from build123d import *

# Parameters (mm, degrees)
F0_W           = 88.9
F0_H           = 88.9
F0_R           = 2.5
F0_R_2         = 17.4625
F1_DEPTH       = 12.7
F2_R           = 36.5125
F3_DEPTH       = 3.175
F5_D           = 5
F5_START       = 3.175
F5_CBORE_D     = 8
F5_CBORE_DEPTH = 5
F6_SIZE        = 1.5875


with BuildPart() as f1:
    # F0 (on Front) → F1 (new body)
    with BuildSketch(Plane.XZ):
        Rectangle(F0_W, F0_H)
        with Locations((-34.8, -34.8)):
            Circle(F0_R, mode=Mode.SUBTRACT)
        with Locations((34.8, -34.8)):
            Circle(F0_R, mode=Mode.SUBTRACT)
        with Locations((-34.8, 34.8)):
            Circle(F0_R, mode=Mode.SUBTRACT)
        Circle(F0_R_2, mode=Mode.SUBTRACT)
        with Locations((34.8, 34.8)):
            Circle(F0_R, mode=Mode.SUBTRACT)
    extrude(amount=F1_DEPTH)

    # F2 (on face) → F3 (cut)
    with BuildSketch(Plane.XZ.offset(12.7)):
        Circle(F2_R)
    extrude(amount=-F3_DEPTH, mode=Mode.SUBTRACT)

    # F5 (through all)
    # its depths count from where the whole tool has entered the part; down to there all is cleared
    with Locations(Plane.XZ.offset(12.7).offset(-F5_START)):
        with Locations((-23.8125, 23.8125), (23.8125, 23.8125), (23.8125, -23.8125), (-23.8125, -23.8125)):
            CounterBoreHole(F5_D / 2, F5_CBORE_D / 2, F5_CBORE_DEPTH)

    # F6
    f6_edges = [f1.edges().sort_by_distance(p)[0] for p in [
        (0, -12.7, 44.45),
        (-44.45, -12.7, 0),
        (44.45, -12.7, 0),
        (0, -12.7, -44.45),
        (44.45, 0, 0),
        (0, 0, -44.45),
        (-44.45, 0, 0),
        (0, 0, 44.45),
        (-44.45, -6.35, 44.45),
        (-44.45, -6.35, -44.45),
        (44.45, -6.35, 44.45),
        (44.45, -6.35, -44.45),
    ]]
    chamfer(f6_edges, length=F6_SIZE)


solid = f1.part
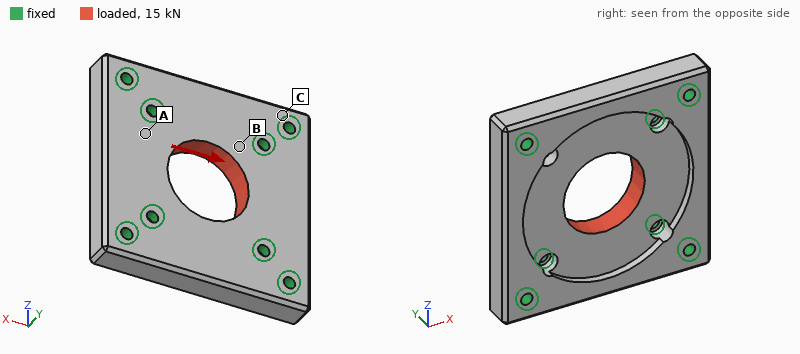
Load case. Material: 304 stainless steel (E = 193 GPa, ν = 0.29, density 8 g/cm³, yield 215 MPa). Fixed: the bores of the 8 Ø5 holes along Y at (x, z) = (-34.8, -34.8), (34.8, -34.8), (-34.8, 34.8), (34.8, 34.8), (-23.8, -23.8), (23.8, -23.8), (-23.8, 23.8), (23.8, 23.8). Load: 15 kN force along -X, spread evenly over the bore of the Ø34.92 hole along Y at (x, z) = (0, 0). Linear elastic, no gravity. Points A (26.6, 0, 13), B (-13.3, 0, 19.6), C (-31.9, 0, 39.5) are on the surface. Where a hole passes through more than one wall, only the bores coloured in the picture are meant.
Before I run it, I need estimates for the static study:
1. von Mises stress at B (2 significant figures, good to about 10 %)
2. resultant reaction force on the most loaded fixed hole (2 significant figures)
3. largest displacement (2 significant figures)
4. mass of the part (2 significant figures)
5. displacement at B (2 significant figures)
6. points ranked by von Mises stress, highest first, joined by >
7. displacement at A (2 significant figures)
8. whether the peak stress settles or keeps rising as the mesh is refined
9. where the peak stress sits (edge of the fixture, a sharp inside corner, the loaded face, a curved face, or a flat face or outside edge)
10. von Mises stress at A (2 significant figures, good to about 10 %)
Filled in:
22 MPa
2.5 kN
3.7 µm
600 g
1.5 µm
B > A > C
1.9 µm
keeps rising
edge of the fixture
13 MPa
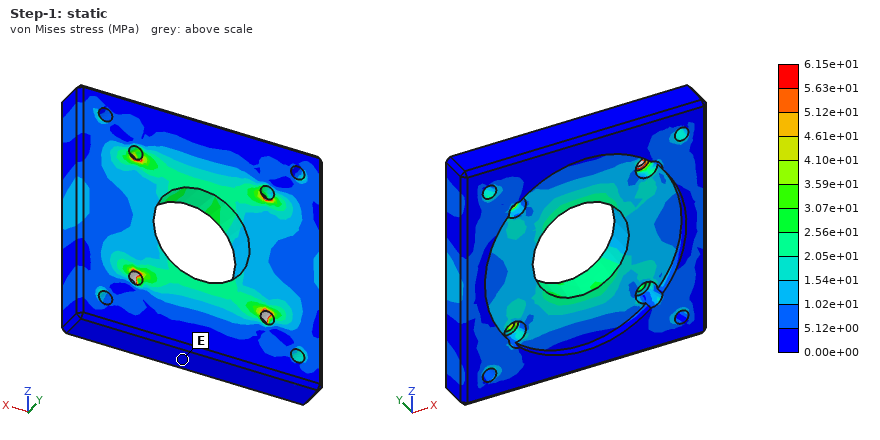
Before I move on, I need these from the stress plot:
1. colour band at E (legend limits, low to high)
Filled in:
0.00e+00 to 5.12e+00 MPa
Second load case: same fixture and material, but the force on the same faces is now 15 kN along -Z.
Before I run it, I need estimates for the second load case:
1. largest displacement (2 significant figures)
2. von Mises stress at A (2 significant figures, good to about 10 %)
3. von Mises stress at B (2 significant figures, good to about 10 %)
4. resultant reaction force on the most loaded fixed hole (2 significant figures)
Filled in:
3.7 µm
15 MPa
14 MPa
2.5 kN
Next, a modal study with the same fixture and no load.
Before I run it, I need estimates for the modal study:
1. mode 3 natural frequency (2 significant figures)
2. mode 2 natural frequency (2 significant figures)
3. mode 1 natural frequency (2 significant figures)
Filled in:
13 kHz
13 kHz
12 kHz
